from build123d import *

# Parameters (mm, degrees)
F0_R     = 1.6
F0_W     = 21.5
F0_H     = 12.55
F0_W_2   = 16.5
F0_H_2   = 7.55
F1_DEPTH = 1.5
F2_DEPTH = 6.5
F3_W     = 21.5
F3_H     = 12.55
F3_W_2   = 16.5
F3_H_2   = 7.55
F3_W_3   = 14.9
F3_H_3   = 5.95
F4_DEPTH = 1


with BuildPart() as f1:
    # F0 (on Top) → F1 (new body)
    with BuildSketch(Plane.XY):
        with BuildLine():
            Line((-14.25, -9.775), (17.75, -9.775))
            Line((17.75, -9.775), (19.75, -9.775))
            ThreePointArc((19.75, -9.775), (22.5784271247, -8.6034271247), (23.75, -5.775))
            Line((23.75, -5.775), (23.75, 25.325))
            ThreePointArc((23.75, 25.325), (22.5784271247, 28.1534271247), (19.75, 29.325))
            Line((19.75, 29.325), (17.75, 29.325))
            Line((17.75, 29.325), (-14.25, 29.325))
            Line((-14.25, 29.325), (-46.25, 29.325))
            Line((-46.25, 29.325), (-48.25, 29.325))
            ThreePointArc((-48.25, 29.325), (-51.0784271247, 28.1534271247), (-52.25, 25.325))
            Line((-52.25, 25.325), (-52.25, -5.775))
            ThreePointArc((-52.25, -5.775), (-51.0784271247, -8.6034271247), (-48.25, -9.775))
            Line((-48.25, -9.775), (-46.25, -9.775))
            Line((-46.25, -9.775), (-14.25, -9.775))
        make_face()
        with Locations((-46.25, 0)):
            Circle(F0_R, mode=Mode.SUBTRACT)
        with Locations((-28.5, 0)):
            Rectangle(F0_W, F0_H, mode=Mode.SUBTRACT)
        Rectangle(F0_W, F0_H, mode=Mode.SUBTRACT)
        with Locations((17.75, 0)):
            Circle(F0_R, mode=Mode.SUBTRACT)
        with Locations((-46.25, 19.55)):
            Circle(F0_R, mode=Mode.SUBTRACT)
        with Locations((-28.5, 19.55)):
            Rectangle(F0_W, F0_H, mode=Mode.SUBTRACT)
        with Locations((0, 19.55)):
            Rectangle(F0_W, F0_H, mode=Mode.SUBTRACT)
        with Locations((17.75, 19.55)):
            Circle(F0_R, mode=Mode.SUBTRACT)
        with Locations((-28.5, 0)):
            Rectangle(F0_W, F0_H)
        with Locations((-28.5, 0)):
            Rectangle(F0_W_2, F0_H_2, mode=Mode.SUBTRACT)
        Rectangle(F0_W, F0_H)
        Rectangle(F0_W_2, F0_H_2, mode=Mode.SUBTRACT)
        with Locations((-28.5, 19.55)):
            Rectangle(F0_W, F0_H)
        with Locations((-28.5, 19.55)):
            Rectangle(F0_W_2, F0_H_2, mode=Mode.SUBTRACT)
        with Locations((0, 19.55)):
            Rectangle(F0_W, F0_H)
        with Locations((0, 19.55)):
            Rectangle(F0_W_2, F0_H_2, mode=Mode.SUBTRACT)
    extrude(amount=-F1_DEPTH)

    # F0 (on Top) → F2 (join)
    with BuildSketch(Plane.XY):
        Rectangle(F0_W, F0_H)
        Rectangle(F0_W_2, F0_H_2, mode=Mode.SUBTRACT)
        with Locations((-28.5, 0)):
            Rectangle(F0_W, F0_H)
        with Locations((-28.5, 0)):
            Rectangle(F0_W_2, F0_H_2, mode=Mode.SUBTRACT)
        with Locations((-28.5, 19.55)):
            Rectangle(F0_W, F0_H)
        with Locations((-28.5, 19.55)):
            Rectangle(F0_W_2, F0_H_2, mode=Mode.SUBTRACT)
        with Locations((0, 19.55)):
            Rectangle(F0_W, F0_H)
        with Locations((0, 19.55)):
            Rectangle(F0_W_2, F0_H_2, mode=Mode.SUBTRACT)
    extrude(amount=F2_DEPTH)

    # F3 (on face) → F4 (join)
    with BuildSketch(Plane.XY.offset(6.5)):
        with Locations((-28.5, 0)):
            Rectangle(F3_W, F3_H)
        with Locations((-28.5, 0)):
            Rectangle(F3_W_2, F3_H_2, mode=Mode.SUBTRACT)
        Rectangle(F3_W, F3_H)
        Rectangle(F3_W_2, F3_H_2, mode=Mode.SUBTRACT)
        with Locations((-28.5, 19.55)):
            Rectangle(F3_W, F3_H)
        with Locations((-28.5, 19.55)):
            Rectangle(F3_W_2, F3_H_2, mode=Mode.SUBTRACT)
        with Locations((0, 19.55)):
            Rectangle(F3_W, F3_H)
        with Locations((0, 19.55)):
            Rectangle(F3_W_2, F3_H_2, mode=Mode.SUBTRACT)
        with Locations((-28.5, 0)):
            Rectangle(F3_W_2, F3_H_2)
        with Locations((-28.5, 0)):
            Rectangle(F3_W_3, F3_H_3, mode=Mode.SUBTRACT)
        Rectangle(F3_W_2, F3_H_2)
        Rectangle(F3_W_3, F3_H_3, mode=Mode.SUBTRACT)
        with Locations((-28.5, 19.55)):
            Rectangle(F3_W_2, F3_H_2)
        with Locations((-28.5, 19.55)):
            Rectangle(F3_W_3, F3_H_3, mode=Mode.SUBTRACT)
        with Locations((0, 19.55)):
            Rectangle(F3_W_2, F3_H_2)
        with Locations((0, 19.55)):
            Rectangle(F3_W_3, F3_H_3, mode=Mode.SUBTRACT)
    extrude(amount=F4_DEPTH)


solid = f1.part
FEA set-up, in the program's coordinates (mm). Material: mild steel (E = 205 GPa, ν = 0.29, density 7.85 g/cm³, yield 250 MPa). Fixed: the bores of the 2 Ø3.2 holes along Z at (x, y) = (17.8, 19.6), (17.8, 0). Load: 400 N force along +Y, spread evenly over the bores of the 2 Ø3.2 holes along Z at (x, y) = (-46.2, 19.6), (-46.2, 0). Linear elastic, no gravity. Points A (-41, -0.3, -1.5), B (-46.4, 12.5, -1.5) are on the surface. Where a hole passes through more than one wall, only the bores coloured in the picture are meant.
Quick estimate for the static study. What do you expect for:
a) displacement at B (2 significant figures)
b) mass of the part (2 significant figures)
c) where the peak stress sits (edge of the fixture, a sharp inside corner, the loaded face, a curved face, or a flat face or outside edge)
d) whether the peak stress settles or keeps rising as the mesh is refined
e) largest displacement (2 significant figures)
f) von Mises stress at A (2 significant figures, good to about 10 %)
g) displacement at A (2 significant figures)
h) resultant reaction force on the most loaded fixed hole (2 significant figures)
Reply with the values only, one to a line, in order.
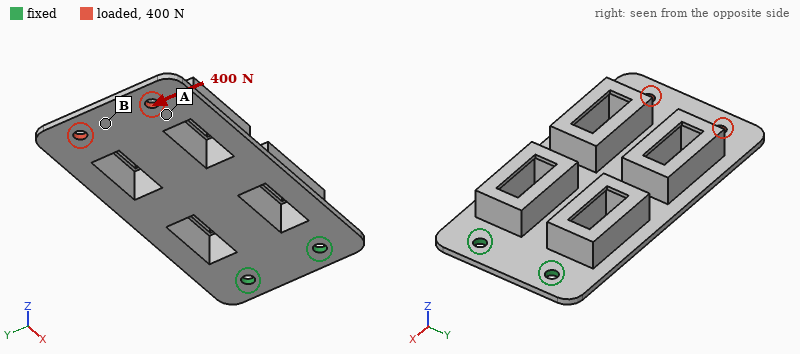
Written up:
56 µm
64 g
edge of the fixture
keeps rising
67 µm
28 MPa
53 µm
1.2 kN
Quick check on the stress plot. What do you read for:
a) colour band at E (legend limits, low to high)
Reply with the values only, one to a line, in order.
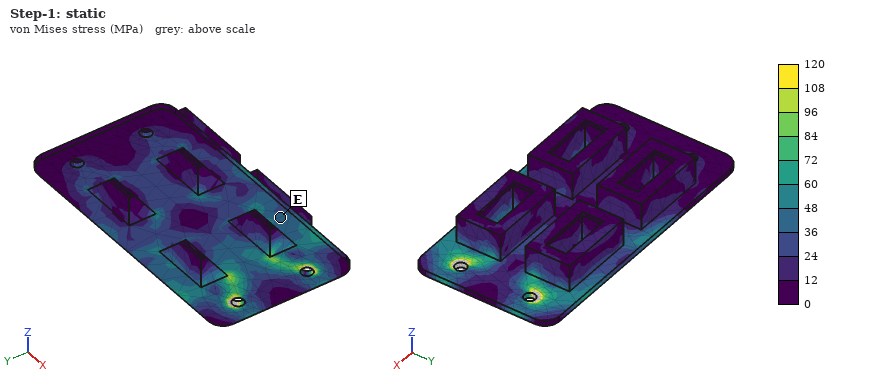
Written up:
36 to 48 MPa
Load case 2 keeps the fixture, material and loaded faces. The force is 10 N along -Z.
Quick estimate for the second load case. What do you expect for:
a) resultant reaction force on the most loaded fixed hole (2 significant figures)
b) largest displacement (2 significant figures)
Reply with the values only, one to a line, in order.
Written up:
5.0 N
0.19 mm
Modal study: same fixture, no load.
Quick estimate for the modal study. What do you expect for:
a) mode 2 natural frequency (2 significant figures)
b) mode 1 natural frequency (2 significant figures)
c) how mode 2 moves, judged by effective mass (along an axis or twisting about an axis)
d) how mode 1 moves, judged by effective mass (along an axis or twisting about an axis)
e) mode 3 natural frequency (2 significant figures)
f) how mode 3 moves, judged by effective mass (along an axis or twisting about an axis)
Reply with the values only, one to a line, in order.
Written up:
1600 Hz
290 Hz
twisting about X
along Z
1800 Hz
along Z
